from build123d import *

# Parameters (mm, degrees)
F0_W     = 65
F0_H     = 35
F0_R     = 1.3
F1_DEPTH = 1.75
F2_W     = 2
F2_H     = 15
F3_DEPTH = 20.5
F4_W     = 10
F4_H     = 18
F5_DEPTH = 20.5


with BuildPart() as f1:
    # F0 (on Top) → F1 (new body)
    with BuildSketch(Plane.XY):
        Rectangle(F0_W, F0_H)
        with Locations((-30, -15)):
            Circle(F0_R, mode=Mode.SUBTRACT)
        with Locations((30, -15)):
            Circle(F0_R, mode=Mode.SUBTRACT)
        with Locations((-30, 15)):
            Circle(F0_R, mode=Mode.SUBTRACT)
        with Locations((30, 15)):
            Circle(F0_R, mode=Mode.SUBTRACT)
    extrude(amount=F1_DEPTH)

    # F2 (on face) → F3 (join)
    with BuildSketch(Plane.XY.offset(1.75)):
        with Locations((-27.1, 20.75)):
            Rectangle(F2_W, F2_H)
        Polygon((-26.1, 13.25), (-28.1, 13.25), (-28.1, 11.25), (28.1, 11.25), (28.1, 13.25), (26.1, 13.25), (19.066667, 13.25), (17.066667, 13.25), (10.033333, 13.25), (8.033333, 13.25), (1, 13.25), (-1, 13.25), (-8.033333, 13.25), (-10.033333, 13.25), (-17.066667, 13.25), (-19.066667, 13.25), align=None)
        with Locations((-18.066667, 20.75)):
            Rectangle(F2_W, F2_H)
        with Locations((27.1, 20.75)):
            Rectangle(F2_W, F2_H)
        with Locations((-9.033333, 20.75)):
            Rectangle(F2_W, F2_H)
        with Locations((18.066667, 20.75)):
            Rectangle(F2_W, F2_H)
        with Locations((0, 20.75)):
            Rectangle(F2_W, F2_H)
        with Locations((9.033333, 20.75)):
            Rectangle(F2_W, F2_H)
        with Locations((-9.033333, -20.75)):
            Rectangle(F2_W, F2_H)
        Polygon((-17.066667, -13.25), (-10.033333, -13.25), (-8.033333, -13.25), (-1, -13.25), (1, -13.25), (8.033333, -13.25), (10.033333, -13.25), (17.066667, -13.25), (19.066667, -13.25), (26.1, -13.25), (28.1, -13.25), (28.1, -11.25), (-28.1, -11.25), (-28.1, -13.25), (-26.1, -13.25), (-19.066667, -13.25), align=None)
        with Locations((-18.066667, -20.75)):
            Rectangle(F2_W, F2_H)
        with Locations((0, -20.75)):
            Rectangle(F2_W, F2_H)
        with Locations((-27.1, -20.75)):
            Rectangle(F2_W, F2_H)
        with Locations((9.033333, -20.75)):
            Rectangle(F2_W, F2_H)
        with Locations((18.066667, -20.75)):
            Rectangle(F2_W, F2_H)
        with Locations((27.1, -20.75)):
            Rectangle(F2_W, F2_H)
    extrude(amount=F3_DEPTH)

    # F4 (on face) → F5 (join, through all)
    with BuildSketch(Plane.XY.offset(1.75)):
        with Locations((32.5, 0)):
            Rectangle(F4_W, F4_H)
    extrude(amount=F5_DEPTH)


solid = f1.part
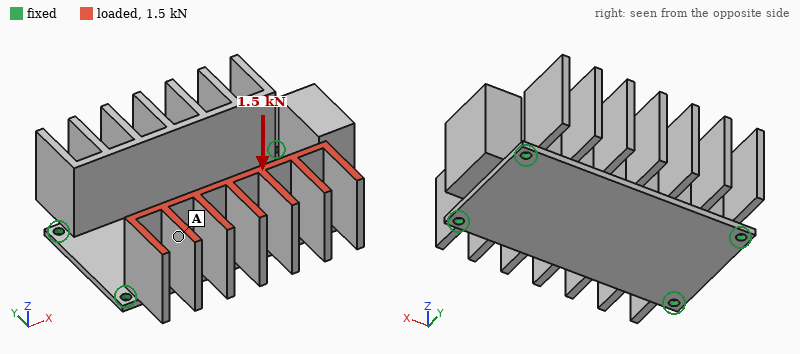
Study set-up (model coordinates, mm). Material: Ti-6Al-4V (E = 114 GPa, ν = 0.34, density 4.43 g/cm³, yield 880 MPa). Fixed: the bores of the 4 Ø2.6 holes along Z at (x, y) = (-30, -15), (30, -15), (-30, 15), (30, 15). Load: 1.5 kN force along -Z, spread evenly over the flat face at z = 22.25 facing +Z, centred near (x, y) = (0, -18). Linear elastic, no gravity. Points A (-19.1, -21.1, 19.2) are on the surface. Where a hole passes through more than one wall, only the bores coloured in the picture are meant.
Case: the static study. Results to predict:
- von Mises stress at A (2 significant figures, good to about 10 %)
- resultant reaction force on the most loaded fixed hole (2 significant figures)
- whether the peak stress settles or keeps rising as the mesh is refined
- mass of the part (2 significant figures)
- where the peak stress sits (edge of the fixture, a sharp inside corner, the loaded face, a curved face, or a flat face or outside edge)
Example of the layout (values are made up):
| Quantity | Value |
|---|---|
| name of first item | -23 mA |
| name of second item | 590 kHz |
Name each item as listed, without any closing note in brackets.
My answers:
| Quantity | Value |
|---|---|
| von Mises stress at A | 14 MPa |
| resultant reaction force on the most loaded fixed hole | 900 N |
| whether the peak stress settles or keeps rising as the mesh is refined | keeps rising |
| mass of the part | 92 g |
| where the peak stress sits | edge of the fixture |
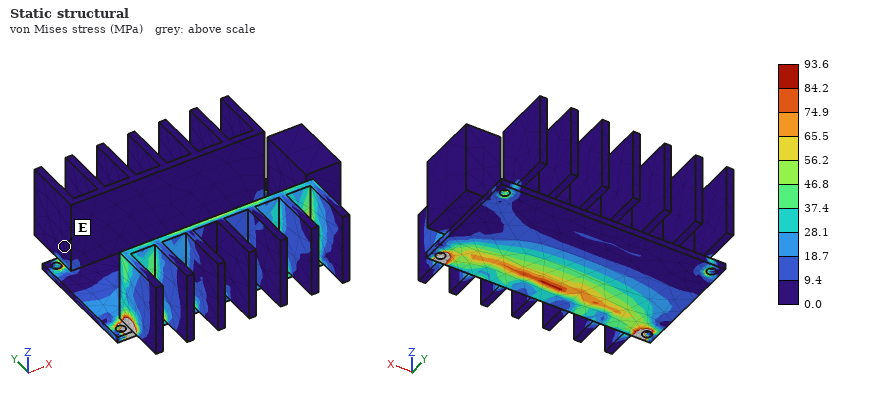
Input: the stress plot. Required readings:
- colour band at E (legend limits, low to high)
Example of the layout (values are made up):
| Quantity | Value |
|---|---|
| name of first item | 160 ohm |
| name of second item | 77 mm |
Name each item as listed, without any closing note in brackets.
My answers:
| Quantity | Value |
|---|---|
| colour band at E | 0.0 to 9.4 MPa |
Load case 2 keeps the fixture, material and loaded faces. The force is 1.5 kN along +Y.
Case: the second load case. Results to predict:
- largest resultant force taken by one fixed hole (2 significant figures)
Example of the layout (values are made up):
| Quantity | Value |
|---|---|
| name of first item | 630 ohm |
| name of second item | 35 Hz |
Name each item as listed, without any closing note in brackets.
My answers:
| Quantity | Value |
|---|---|
| largest resultant force taken by one fixed hole | 750 N |
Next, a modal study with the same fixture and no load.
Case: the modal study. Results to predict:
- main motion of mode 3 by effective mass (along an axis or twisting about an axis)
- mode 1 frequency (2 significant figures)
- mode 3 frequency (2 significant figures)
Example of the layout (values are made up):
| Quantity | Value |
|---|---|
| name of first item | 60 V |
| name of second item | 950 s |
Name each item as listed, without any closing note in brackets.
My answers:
| Quantity | Value |
|---|---|
| main motion of mode 3 by effective mass | along Y |
| mode 1 frequency | 1800 Hz |
| mode 3 frequency | 2500 Hz |
